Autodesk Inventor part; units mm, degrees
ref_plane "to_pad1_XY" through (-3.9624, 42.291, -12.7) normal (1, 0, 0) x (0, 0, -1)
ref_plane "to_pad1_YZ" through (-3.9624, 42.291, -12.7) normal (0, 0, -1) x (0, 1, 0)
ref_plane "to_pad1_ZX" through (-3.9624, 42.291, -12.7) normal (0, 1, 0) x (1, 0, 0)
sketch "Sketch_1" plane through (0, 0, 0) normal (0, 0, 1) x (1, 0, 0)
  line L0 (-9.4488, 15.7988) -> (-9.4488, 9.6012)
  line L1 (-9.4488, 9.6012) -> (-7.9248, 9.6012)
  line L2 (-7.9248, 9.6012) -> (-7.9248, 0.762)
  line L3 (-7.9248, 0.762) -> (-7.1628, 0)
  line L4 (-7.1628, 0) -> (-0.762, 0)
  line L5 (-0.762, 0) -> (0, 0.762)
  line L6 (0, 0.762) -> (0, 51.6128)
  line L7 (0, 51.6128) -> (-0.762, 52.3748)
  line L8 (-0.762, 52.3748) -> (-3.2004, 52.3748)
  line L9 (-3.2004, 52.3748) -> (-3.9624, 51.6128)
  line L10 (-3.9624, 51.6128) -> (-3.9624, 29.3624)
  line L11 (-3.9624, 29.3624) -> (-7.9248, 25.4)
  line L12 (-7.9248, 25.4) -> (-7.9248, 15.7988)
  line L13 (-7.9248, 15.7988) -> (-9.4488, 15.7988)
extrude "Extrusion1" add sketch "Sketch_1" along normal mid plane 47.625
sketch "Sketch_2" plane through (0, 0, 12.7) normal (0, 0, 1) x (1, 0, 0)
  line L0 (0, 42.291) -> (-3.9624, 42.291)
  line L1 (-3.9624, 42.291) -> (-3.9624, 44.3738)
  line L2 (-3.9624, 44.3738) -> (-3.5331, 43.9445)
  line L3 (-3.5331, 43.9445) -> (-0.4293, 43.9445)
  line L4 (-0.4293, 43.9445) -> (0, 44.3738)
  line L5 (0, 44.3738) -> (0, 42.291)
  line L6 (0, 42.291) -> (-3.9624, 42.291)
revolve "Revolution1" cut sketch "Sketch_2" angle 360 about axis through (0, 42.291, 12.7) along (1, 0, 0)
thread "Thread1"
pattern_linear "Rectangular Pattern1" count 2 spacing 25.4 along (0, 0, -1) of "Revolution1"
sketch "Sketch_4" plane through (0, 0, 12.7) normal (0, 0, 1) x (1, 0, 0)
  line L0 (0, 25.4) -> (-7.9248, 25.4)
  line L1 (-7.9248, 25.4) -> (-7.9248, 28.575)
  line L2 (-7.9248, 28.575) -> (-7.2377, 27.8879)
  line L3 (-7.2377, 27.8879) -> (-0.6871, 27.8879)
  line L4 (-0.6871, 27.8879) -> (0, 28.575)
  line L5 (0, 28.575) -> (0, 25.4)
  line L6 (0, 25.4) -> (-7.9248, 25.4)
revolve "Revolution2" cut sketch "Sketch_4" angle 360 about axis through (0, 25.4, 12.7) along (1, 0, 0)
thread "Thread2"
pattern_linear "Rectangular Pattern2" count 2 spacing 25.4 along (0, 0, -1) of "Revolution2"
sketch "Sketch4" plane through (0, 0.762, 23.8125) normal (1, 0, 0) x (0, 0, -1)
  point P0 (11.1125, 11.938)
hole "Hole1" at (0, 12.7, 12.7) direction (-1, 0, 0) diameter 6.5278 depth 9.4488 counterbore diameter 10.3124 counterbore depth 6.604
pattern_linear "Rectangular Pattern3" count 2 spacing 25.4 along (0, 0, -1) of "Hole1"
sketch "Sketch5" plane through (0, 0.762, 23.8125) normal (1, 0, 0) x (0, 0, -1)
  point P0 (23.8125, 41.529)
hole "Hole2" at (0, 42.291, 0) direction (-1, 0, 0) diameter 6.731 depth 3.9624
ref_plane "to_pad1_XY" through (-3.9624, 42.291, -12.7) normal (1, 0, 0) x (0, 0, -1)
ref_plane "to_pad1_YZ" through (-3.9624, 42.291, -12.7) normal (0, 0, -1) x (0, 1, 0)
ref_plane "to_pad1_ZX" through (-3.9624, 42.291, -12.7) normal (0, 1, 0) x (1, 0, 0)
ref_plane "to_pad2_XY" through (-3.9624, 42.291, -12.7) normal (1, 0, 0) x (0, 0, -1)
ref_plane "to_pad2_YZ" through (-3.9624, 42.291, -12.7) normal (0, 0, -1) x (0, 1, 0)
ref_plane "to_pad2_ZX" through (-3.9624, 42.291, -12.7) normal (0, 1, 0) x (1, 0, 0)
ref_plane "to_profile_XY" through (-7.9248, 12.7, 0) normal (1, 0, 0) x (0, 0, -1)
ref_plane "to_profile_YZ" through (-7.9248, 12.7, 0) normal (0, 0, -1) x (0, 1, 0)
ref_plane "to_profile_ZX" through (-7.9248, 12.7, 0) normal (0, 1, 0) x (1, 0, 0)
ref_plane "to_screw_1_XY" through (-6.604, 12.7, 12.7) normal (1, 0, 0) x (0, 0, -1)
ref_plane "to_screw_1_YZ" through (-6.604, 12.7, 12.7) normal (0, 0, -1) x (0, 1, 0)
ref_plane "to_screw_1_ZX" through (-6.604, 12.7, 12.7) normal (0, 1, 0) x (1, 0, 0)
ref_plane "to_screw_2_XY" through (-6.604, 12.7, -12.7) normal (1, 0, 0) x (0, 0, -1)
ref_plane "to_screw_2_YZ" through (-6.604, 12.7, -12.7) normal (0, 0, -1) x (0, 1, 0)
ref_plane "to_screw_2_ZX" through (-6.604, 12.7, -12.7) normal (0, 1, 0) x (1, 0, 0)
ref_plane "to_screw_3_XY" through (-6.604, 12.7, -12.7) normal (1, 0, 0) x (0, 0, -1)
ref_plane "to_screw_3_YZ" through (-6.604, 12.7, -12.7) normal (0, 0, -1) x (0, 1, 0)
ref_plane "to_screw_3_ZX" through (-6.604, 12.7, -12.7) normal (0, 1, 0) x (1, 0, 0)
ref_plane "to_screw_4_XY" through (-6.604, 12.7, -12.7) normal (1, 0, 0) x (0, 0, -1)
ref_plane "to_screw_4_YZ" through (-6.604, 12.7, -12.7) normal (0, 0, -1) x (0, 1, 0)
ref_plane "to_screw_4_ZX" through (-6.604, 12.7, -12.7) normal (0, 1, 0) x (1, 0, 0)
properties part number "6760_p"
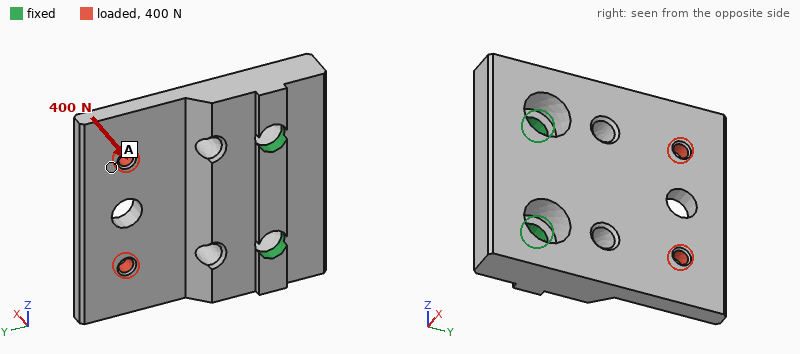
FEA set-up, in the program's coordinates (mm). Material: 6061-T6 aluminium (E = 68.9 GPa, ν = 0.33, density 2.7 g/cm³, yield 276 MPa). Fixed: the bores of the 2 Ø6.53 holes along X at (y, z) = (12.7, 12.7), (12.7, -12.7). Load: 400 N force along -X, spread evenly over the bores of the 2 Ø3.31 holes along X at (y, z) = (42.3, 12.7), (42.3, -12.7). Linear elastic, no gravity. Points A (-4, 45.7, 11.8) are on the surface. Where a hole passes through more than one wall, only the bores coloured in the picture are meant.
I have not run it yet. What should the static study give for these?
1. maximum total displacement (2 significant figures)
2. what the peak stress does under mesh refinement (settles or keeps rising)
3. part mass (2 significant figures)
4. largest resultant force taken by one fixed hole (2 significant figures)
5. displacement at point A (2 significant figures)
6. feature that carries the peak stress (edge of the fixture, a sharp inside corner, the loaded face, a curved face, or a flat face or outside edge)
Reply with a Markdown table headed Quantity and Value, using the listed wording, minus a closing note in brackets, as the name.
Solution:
| Quantity | Value |
|---|---|
| maximum total displacement | 0.20 mm |
| what the peak stress does under mesh refinement | keeps rising |
| part mass | 37 g |
| largest resultant force taken by one fixed hole | 240 N |
| displacement at point A | 0.16 mm |
| feature that carries the peak stress | edge of the fixture |
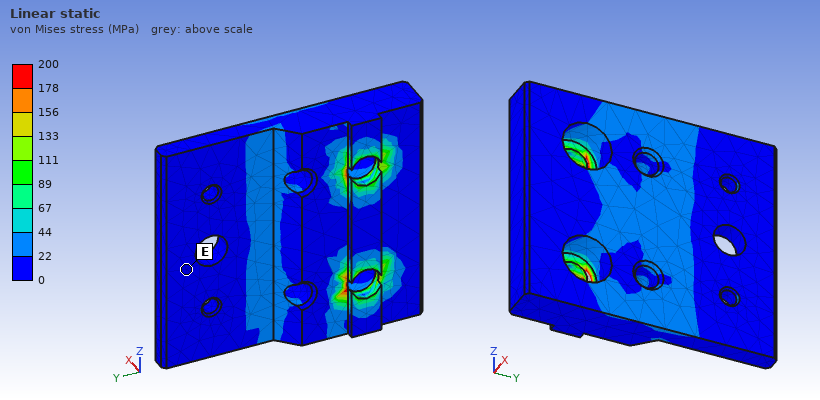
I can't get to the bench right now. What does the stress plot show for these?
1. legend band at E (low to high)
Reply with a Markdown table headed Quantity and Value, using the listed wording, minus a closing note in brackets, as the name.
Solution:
| Quantity | Value |
|---|---|
| legend band at E | 0 to 22 MPa |
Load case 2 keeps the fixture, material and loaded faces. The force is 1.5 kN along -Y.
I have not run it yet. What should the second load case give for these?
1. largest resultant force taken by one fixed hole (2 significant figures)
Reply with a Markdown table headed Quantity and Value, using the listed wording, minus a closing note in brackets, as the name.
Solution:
| Quantity | Value |
|---|---|
| largest resultant force taken by one fixed hole | 750 N |
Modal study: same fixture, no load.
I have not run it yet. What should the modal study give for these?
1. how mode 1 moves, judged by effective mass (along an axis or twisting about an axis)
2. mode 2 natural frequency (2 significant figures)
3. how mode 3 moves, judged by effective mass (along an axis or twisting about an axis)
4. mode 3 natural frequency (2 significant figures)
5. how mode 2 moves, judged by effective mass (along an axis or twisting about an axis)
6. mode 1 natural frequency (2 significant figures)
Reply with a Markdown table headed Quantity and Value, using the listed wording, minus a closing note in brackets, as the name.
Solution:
| Quantity | Value |
|---|---|
| how mode 1 moves, judged by effective mass | along X |
| mode 2 natural frequency | 5500 Hz |
| how mode 3 moves, judged by effective mass | along Y |
| mode 3 natural frequency | 9300 Hz |
| how mode 2 moves, judged by effective mass | twisting about Y |
| mode 1 natural frequency | 2500 Hz |
